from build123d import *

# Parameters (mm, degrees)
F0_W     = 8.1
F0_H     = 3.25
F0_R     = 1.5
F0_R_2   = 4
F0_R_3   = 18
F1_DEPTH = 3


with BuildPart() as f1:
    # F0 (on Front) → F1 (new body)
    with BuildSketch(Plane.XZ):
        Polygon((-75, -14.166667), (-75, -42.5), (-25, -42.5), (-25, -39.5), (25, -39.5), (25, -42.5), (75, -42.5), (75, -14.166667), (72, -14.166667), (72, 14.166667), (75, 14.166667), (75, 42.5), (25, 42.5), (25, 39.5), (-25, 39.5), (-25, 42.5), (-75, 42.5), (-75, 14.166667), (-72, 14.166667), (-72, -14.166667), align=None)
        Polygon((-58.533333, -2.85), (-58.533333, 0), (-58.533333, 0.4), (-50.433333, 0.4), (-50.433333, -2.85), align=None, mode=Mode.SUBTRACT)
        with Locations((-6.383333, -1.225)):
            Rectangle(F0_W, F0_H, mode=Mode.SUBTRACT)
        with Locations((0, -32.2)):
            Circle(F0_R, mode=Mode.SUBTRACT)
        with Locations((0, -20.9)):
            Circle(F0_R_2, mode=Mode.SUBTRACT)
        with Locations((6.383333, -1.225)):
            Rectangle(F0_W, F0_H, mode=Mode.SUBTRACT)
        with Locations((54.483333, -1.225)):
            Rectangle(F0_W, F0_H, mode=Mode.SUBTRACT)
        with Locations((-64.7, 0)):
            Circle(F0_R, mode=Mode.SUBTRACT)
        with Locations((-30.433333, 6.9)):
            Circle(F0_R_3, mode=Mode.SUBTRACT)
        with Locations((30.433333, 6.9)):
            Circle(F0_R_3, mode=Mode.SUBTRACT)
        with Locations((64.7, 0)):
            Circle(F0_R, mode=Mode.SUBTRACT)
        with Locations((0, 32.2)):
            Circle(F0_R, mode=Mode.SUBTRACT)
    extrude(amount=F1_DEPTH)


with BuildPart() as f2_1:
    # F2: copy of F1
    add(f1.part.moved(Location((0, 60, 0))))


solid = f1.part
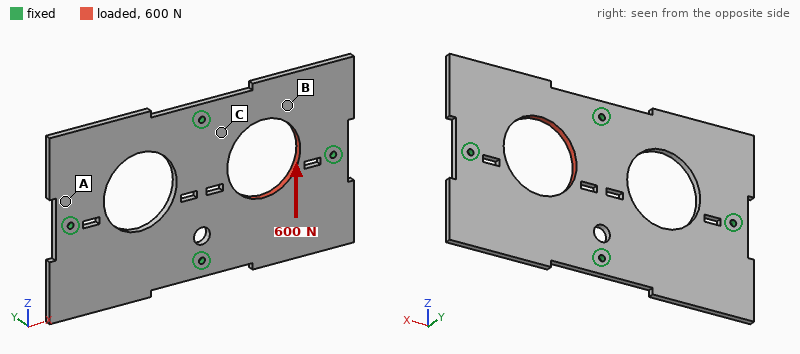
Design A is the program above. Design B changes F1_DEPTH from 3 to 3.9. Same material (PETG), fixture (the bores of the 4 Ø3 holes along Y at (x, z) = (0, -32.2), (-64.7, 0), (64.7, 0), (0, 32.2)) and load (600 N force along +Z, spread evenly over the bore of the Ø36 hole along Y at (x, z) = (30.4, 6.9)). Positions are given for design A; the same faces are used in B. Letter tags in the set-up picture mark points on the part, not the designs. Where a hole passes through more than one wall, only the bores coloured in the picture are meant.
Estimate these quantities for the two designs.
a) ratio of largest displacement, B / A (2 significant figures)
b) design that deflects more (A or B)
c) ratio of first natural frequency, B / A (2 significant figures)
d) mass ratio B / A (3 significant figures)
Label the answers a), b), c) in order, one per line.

a) 0.77
b) A
c) 1.3
d) 1.30
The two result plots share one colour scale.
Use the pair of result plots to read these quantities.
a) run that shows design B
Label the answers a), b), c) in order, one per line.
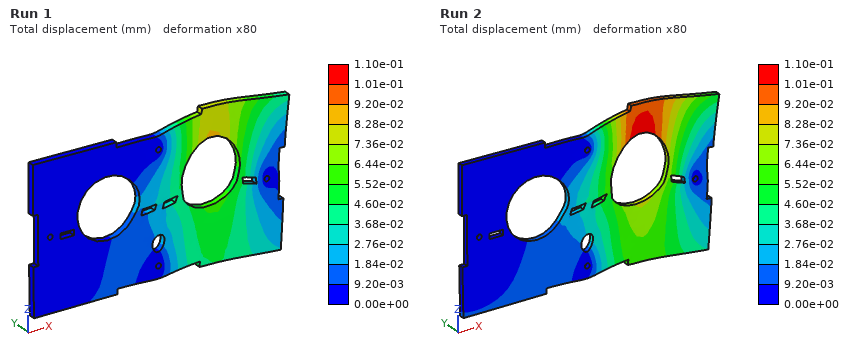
a) Run 1
